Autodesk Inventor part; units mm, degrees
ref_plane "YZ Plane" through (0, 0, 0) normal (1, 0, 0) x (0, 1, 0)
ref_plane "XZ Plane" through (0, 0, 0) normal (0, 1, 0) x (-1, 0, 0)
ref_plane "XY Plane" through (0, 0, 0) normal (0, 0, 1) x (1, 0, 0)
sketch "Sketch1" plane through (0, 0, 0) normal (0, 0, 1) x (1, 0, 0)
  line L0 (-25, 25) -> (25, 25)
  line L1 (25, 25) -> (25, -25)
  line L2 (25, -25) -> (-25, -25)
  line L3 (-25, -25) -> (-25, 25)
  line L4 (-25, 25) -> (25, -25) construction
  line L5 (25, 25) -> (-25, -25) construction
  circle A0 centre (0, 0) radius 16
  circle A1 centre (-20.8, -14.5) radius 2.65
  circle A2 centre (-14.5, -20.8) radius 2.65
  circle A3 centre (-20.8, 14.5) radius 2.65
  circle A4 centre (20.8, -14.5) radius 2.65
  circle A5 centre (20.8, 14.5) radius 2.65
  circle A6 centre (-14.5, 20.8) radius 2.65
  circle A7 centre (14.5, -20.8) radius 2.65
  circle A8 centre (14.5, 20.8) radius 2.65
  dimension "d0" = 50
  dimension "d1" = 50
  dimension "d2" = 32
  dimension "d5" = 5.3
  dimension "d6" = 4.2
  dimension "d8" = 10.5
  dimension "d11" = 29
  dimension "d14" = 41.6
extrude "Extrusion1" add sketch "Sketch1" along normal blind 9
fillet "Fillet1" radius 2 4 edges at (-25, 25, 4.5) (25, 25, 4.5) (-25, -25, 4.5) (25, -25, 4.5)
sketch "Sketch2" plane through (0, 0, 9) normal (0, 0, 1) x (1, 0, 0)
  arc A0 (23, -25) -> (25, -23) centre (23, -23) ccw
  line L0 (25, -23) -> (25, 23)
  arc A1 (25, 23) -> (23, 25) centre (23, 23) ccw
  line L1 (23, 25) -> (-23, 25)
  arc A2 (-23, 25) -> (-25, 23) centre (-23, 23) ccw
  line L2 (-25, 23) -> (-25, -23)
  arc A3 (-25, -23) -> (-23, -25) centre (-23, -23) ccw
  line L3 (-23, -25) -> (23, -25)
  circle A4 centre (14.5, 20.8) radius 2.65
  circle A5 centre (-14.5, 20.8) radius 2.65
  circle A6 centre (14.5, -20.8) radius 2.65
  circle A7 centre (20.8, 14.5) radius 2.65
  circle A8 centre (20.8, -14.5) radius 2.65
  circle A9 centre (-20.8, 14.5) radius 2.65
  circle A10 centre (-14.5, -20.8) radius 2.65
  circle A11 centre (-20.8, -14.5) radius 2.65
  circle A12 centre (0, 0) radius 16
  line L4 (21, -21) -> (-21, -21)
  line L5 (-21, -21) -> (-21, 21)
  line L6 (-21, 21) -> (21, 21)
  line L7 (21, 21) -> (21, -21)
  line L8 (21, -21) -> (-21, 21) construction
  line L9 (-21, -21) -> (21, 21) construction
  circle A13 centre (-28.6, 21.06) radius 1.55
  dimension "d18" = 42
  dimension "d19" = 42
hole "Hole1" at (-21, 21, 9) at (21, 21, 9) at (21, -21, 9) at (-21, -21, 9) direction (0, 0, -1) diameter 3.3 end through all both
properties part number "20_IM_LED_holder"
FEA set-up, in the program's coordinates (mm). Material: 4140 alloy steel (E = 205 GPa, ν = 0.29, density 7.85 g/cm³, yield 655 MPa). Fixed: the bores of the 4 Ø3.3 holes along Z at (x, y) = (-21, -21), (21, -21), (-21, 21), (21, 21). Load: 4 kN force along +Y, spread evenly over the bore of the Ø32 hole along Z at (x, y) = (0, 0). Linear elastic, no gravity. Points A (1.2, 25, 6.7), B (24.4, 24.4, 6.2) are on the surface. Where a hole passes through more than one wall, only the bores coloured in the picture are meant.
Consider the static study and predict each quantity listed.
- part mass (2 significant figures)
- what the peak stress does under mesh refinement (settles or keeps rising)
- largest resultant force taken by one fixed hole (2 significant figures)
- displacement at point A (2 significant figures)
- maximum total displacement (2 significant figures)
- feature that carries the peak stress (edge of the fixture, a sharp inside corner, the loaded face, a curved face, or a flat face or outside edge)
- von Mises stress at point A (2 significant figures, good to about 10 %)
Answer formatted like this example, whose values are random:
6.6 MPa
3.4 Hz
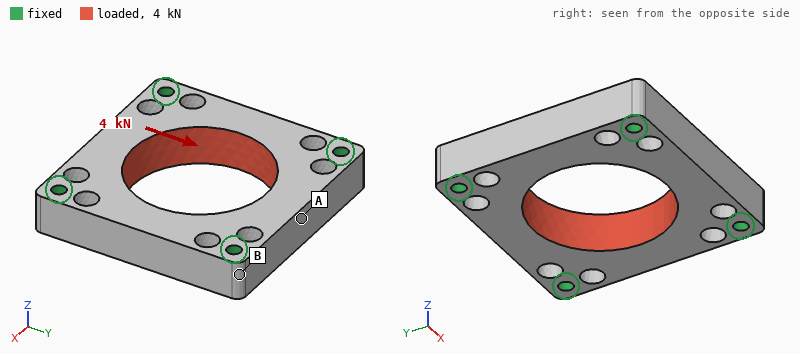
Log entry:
100 g
keeps rising
1.0 kN
2.9 µm
3.1 µm
edge of the fixture
15 MPa
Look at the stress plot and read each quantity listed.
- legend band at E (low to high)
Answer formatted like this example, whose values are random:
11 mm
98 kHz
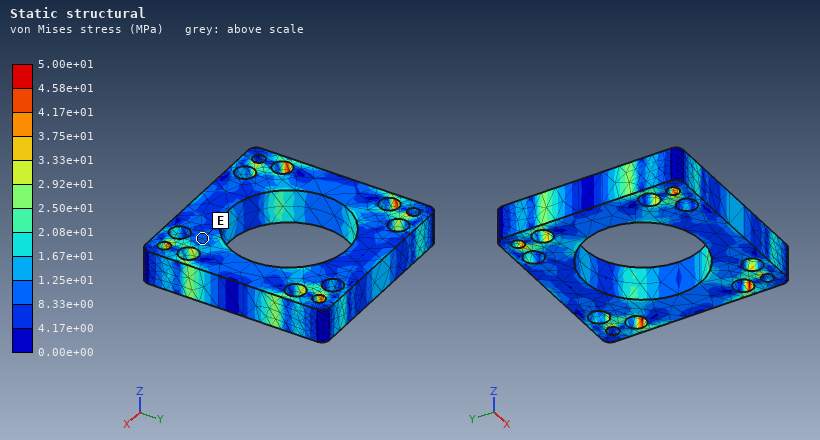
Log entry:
8.33e+00 to 1.25e+01 MPa
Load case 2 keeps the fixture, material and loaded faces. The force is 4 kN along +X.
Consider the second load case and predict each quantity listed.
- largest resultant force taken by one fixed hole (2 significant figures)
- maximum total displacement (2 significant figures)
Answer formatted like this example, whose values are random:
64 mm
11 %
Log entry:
1.0 kN
3.1 µm
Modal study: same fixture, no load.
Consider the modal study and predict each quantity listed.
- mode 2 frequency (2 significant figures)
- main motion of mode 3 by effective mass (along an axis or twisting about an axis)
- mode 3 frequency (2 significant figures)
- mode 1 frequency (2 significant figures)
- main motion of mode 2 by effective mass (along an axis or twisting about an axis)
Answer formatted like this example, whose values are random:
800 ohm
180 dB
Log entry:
17 kHz
twisting about X
19 kHz
15 kHz
along Z
